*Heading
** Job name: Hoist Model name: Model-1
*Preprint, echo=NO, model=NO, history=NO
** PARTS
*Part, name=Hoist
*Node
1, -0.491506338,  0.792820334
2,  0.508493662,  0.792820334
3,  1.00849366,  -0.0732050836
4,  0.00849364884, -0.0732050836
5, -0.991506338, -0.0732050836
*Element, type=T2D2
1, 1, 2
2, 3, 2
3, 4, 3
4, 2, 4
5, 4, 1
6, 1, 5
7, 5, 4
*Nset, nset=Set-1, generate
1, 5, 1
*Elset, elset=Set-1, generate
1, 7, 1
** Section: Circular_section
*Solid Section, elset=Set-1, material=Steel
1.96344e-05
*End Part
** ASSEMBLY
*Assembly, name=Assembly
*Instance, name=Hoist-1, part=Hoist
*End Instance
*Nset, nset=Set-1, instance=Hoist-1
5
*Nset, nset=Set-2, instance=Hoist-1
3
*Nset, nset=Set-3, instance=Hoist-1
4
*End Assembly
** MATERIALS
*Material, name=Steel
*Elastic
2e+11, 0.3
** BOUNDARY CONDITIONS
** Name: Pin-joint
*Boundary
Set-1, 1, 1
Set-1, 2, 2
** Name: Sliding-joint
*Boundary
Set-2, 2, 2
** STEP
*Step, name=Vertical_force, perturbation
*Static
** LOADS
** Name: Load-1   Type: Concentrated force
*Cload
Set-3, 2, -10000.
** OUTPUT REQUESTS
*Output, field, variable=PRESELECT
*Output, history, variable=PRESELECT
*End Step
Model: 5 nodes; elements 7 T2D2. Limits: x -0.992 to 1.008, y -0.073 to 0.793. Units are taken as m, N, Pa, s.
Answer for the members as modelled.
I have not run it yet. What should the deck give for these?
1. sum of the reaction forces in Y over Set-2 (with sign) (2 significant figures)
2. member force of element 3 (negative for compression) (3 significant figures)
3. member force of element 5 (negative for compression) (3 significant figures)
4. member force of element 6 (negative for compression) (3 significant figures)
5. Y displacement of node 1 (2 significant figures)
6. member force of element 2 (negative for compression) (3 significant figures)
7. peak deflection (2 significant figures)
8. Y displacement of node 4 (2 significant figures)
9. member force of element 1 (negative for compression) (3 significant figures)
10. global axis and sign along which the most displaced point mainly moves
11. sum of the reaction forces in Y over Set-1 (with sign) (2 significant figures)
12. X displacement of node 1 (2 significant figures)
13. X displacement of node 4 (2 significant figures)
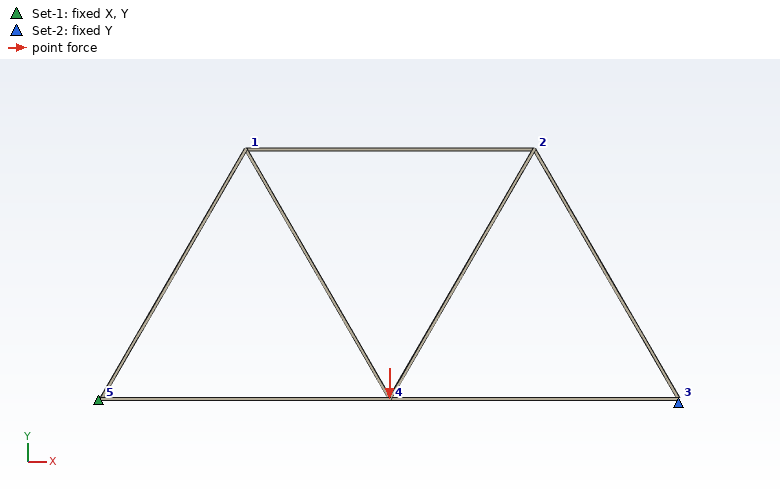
5000 N
2890 N
5770 N
-5770 N
-0.0025 m
-5770 N
0.0047 m
-0.0047 m
-5770 N
-Y
5000 N
0.0015 m
7.4e-04 m
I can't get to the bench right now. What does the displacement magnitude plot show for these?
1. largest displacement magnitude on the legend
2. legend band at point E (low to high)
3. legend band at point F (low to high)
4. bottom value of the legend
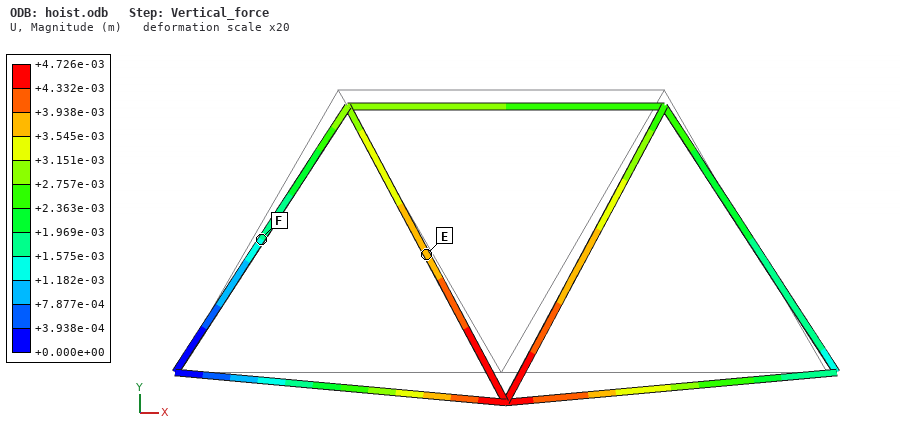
+4.726e-03 m
+3.545e-03 to +3.938e-03 m
+1.182e-03 to +1.575e-03 m
+0.000e+00 m
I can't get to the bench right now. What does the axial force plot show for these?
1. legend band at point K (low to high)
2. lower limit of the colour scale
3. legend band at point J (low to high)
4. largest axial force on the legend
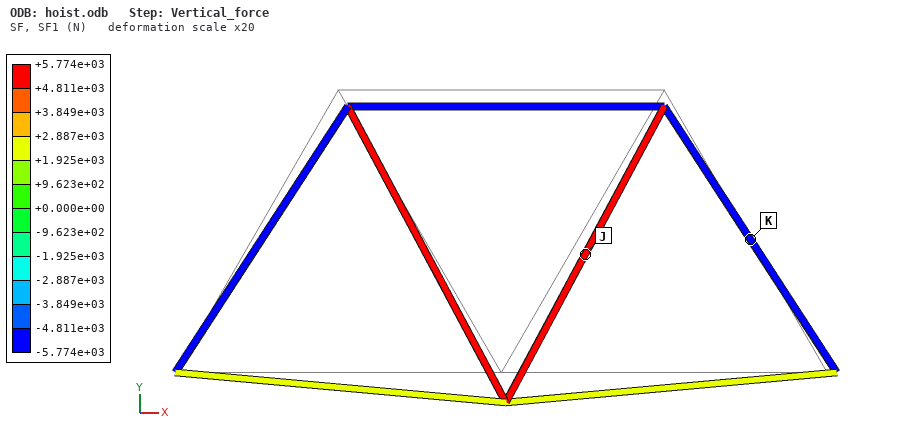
-5.774e+03 to -4.811e+03 N
-5.774e+03 N
+4.811e+03 to +5.774e+03 N
+5.774e+03 N
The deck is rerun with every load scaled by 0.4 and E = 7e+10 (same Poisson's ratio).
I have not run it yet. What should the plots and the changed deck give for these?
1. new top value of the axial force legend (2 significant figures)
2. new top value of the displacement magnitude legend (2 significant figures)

2300 N
0.0054 m
